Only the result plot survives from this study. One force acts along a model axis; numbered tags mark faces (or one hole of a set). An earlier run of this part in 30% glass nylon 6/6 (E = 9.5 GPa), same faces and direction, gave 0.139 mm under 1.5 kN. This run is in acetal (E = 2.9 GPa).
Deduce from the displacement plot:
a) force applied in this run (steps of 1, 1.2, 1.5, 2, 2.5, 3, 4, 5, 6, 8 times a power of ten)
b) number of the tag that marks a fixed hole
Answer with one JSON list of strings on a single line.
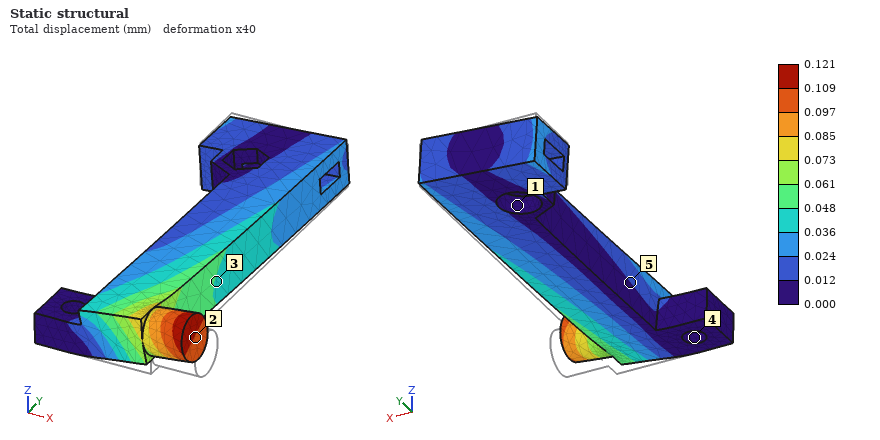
["400 N", "4"]
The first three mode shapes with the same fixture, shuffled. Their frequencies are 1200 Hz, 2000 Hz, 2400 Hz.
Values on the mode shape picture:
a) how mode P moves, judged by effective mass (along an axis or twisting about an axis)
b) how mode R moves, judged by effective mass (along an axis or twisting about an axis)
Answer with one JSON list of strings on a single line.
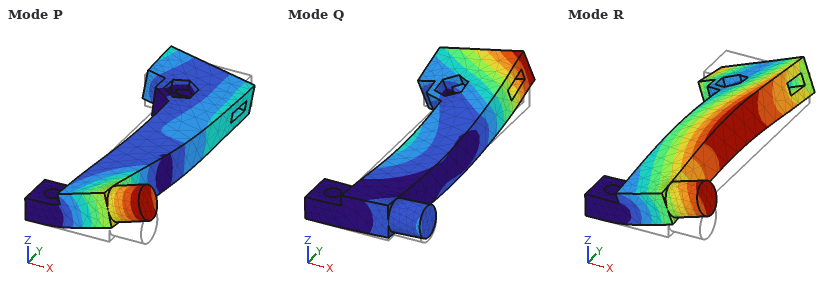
["twisting about X", "along Z"]
